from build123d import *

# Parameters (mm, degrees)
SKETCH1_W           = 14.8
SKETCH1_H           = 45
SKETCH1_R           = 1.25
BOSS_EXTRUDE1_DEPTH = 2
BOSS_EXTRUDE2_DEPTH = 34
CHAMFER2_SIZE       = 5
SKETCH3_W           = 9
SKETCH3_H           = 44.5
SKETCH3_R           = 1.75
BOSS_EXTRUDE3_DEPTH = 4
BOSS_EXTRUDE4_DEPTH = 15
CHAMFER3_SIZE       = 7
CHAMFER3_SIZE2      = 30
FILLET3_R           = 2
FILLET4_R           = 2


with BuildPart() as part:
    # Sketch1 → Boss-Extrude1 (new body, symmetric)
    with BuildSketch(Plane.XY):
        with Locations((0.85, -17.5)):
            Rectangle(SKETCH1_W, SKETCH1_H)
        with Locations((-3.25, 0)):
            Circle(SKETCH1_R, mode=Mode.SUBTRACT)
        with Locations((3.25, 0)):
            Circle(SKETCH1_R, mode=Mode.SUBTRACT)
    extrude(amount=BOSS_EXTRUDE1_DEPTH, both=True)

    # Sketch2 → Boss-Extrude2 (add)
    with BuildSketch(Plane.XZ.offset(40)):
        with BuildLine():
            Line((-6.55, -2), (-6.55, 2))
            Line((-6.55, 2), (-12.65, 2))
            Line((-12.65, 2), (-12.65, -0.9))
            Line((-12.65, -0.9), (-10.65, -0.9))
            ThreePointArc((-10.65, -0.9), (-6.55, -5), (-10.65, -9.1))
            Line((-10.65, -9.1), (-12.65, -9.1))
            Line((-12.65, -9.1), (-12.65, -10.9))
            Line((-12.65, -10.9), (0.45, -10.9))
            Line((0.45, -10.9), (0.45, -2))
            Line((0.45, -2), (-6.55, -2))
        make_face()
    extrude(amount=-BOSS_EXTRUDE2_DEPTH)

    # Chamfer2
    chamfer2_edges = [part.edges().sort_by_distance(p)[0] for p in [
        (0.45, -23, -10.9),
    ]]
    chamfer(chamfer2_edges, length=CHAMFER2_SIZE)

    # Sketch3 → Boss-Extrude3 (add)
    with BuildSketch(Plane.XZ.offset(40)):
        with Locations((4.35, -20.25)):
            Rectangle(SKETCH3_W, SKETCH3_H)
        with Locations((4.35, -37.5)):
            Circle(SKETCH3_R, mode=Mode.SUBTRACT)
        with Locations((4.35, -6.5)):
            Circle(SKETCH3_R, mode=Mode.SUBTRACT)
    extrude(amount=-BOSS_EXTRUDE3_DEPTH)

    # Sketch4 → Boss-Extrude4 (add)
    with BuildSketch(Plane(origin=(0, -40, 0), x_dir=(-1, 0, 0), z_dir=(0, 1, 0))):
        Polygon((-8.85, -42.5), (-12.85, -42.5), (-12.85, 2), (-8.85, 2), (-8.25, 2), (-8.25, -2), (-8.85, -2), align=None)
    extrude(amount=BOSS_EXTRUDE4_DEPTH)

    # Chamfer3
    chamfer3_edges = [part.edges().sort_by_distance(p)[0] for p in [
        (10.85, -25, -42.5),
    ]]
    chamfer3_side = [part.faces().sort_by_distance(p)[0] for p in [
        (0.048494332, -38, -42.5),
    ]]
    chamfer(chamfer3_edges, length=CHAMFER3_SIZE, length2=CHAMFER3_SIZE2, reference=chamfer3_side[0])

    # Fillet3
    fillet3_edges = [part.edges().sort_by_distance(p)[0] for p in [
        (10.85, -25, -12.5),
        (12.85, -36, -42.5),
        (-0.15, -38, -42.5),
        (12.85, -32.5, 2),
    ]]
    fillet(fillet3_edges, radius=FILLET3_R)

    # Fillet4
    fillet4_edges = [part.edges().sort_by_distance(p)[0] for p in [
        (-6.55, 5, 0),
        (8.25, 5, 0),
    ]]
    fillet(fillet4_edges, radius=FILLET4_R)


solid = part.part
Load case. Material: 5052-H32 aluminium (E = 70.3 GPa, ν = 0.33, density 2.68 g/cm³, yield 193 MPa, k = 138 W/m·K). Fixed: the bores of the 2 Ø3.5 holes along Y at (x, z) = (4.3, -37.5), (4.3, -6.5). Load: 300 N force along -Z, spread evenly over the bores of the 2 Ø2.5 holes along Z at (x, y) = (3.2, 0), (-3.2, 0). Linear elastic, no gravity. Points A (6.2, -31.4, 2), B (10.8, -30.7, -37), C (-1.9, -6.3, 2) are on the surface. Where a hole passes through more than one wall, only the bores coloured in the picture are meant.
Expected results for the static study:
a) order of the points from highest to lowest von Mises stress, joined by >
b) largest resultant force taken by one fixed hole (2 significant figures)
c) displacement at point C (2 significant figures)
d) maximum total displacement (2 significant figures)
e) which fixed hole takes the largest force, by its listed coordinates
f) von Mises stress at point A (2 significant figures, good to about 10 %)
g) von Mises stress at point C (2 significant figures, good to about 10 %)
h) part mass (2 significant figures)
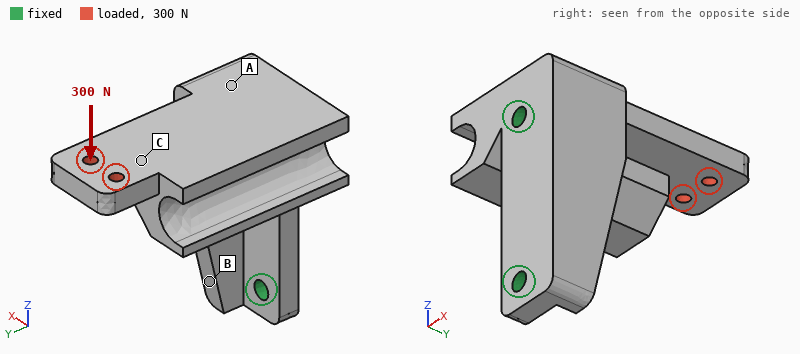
A > C > B
300 N
0.19 mm
0.29 mm
(4.3, -37.5)
69 MPa
42 MPa
25 g
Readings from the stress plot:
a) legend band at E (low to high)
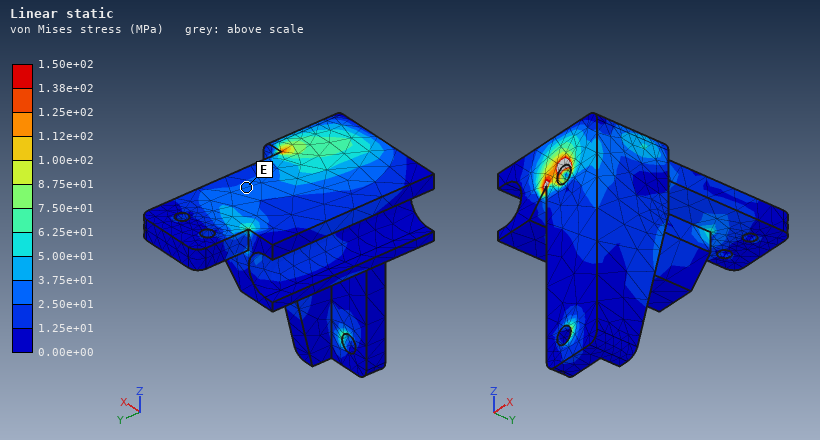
2.50e+01 to 3.75e+01 MPa
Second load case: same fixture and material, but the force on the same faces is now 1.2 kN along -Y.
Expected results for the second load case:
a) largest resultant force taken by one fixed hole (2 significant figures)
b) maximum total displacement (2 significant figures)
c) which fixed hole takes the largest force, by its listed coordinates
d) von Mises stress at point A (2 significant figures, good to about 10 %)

1.3 kN
0.15 mm
(4.3, -6.5)
29 MPa
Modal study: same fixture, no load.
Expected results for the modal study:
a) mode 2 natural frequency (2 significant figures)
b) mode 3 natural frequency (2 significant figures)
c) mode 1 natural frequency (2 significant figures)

2900 Hz
8400 Hz
2500 Hz
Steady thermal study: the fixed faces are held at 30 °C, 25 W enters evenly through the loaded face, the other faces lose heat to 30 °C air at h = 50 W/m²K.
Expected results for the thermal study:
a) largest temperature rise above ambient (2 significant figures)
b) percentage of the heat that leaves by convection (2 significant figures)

75 K
22 %
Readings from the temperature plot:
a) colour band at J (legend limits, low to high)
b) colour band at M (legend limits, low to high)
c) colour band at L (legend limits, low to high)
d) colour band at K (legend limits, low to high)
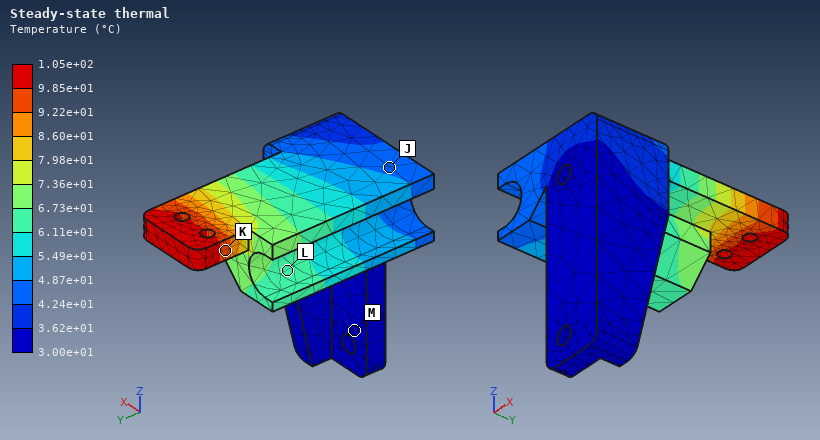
4.24e+01 to 4.87e+01 °C
3.00e+01 to 3.62e+01 °C
6.11e+01 to 6.73e+01 °C
9.22e+01 to 9.85e+01 °C
